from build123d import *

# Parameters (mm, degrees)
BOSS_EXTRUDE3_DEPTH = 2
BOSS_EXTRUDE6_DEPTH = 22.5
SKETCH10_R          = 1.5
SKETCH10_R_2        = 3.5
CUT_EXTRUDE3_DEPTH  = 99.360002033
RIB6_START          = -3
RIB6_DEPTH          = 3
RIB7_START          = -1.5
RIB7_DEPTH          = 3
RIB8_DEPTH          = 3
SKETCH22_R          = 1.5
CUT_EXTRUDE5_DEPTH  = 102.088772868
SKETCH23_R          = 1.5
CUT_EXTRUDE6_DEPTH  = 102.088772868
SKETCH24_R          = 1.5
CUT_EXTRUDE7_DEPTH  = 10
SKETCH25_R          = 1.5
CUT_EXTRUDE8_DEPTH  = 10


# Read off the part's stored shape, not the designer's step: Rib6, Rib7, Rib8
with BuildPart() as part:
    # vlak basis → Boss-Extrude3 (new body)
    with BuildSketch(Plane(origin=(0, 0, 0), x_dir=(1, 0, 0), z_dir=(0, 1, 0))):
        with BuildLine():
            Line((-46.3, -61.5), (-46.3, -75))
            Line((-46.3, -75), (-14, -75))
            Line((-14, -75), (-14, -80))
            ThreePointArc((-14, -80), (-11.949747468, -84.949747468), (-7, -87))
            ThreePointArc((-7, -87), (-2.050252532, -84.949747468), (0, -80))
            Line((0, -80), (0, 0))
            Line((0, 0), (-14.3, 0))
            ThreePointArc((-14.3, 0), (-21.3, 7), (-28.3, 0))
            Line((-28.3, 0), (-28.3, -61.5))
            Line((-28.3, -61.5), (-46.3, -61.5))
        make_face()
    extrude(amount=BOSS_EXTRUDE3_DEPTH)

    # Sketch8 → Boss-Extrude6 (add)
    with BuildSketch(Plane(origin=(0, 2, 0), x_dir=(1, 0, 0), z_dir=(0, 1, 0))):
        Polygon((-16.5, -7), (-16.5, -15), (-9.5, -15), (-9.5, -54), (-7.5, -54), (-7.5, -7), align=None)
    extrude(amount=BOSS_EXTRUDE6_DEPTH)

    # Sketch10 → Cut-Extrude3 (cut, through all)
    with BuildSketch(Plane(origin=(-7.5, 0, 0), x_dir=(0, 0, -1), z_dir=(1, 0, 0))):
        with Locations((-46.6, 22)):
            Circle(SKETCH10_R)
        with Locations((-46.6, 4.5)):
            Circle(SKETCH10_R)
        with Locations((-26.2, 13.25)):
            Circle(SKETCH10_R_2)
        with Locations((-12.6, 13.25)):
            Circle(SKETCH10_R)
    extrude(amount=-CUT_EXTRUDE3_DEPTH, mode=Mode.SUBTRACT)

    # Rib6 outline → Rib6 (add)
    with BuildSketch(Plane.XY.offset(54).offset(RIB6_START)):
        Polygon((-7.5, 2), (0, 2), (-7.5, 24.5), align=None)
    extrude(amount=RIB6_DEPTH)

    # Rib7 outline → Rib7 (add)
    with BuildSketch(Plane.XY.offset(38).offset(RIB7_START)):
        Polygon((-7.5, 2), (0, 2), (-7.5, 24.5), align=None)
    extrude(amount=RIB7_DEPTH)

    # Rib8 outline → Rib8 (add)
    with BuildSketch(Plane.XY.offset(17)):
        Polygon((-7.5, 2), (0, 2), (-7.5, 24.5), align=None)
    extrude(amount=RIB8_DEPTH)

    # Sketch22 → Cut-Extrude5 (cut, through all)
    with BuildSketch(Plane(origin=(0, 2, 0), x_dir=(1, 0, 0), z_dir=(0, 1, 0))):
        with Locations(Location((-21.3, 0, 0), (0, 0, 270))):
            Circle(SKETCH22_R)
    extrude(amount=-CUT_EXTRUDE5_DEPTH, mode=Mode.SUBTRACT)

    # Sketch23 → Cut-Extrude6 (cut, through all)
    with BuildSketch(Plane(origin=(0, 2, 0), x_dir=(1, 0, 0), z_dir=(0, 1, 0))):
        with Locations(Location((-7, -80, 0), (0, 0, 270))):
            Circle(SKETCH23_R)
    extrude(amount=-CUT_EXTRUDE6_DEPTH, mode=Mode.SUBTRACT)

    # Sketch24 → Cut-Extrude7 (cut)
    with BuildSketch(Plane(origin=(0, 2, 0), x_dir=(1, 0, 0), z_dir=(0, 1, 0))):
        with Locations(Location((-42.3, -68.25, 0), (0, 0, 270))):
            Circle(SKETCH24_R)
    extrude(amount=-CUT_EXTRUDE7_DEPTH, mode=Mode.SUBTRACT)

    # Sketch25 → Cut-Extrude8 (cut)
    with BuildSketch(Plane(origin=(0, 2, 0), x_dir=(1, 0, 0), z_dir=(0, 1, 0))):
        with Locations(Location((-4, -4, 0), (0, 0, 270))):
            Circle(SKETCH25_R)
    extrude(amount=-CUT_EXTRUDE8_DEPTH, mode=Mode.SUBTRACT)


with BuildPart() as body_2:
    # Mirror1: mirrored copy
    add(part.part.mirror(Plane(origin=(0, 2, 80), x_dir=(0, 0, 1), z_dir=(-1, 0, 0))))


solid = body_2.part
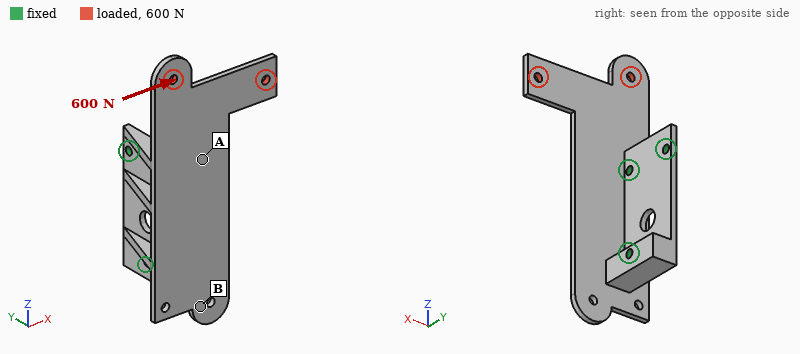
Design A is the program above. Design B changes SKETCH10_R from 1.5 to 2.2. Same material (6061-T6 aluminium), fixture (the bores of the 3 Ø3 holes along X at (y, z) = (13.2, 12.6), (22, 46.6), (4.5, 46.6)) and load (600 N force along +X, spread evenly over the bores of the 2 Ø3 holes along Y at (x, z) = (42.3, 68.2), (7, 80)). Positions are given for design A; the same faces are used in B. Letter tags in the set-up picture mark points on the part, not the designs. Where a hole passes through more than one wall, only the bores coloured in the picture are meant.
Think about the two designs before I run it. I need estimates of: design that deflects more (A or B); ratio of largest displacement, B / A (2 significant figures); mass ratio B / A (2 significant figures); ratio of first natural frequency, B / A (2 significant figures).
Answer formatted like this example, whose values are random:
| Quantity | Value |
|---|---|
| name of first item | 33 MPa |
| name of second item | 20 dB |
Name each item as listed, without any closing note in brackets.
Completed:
| Quantity | Value |
|---|---|
| design that deflects more | A |
| ratio of largest displacement, B / A | 0.82 |
| mass ratio B / A | 0.99 |
| ratio of first natural frequency, B / A | 1.0 |
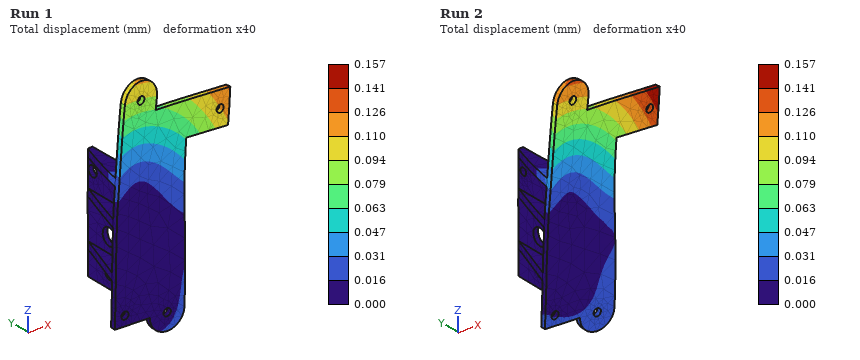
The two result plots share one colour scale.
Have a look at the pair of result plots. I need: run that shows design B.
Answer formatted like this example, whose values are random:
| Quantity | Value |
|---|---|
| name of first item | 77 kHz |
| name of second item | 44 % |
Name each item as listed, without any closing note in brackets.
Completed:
| Quantity | Value |
|---|---|
| run that shows design B | Run 1 |
